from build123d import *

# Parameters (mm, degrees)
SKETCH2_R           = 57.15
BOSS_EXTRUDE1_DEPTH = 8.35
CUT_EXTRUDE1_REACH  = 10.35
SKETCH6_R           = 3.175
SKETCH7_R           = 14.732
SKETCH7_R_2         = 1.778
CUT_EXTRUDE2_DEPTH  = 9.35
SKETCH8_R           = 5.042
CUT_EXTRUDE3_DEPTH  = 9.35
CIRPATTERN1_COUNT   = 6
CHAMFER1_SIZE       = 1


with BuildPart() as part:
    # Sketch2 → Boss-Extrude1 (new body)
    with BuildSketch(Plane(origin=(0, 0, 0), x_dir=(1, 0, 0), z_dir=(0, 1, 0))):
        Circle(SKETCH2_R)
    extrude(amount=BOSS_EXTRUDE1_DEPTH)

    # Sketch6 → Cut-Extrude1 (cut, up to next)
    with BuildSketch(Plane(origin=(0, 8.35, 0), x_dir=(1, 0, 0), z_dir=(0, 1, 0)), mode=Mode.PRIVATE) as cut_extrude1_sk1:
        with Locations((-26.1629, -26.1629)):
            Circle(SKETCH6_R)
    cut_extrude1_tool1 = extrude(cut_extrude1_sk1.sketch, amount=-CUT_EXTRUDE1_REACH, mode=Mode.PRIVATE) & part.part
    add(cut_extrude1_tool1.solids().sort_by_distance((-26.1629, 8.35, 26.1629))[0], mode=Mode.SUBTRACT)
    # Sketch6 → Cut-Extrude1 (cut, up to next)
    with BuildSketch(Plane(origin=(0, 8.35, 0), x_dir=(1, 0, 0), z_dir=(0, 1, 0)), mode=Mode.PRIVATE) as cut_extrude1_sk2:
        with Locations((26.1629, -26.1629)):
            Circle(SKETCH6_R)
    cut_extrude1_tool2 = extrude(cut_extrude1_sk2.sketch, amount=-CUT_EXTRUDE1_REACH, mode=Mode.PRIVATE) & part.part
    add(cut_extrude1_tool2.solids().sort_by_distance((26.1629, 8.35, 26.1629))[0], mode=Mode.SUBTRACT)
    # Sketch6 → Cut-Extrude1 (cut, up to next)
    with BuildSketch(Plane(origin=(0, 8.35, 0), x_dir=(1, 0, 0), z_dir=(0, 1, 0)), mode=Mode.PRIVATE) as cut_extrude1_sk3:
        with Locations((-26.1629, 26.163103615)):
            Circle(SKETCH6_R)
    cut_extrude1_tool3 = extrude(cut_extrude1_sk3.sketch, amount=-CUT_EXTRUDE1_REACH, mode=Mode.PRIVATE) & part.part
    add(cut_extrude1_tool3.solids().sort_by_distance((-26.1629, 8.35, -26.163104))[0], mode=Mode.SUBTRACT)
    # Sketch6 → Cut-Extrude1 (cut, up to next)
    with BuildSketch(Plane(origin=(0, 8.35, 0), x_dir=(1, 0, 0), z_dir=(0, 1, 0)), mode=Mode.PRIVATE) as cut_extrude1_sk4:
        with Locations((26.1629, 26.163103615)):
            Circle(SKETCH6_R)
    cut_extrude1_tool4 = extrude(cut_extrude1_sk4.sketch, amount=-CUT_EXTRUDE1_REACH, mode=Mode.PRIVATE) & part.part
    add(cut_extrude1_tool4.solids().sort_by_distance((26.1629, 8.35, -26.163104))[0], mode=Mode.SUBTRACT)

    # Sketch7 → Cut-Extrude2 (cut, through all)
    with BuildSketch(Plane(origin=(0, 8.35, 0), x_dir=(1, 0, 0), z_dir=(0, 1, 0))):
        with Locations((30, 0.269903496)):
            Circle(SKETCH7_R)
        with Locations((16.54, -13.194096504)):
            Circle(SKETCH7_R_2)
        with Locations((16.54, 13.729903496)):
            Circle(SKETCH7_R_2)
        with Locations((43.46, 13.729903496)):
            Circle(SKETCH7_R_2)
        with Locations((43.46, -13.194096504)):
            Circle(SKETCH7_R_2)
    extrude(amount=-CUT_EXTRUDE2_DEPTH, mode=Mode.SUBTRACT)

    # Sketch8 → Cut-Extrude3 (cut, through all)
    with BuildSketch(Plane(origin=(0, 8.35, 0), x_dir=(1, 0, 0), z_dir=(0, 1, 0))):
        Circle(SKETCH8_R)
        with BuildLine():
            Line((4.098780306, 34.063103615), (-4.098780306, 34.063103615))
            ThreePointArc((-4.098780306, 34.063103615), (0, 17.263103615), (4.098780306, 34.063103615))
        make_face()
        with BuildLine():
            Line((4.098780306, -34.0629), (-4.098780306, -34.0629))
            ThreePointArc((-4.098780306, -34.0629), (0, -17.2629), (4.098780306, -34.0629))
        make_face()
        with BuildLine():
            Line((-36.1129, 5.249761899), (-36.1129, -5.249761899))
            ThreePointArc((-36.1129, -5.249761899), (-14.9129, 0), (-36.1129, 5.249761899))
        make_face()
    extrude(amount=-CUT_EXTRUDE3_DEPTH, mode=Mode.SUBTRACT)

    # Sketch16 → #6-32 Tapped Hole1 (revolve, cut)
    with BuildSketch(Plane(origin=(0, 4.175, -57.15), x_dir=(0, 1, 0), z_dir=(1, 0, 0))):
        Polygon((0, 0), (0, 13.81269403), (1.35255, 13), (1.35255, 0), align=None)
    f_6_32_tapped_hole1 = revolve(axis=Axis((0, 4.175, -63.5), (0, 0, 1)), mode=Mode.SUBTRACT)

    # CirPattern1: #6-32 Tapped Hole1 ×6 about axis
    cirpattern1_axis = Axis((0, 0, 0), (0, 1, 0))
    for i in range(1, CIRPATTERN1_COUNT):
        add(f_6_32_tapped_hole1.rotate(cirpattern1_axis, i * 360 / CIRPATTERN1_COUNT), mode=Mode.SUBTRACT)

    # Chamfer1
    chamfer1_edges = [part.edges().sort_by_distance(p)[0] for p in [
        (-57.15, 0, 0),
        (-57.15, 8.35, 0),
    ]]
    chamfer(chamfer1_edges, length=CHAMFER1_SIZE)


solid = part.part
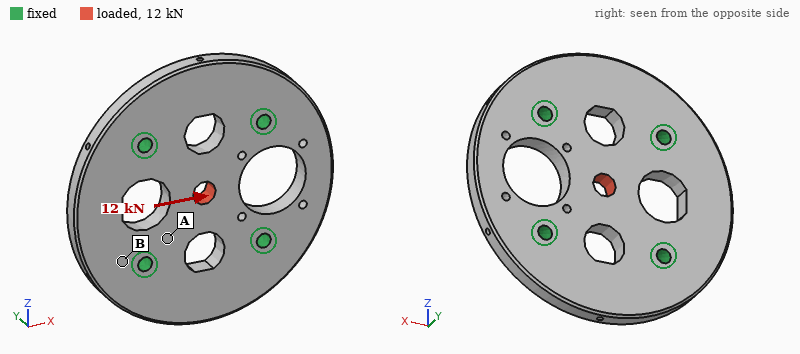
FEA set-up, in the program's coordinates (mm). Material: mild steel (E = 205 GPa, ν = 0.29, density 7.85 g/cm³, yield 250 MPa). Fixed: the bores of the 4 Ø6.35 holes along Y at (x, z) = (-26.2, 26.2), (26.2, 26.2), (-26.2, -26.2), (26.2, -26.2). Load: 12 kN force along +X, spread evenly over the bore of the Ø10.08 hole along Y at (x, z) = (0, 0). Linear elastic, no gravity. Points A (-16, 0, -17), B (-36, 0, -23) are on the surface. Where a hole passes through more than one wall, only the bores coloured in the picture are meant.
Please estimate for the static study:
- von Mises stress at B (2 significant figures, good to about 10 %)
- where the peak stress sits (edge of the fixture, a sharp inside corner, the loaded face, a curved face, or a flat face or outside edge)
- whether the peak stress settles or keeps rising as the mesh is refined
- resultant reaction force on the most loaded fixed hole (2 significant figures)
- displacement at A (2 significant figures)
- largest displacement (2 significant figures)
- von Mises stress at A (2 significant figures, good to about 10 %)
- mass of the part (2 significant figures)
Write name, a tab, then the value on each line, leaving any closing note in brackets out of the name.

von Mises stress at B	10 MPa
where the peak stress sits	a sharp inside corner
whether the peak stress settles or keeps rising as the mesh is refined	keeps rising
resultant reaction force on the most loaded fixed hole	3.7 kN
displacement at A	1.8 µm
largest displacement	7.0 µm
von Mises stress at A	25 MPa
mass of the part	550 g
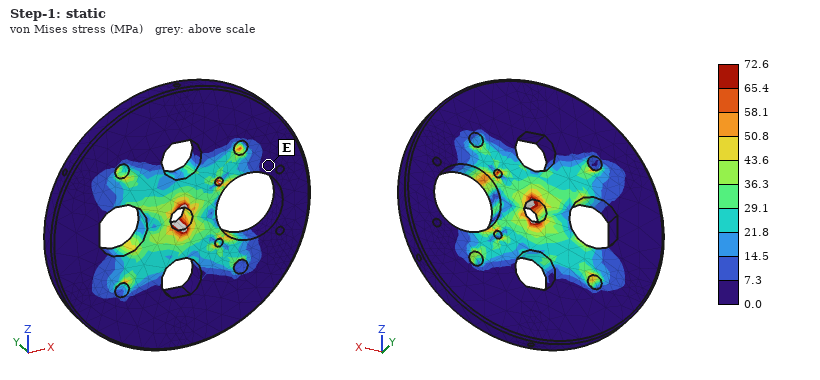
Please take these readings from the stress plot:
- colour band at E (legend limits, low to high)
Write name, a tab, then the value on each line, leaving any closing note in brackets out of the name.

colour band at E	0.0 to 7.3 MPa
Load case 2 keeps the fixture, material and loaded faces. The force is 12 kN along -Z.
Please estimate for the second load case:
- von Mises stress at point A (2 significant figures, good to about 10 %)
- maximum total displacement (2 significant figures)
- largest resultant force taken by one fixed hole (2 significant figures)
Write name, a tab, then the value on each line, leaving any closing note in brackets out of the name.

von Mises stress at point A	24 MPa
maximum total displacement	6.0 µm
largest resultant force taken by one fixed hole	3.4 kN
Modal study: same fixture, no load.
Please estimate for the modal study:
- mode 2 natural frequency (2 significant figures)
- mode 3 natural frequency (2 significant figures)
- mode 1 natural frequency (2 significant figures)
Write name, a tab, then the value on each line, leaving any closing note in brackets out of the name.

mode 2 natural frequency	6700 Hz
mode 3 natural frequency	7000 Hz
mode 1 natural frequency	6200 Hz
